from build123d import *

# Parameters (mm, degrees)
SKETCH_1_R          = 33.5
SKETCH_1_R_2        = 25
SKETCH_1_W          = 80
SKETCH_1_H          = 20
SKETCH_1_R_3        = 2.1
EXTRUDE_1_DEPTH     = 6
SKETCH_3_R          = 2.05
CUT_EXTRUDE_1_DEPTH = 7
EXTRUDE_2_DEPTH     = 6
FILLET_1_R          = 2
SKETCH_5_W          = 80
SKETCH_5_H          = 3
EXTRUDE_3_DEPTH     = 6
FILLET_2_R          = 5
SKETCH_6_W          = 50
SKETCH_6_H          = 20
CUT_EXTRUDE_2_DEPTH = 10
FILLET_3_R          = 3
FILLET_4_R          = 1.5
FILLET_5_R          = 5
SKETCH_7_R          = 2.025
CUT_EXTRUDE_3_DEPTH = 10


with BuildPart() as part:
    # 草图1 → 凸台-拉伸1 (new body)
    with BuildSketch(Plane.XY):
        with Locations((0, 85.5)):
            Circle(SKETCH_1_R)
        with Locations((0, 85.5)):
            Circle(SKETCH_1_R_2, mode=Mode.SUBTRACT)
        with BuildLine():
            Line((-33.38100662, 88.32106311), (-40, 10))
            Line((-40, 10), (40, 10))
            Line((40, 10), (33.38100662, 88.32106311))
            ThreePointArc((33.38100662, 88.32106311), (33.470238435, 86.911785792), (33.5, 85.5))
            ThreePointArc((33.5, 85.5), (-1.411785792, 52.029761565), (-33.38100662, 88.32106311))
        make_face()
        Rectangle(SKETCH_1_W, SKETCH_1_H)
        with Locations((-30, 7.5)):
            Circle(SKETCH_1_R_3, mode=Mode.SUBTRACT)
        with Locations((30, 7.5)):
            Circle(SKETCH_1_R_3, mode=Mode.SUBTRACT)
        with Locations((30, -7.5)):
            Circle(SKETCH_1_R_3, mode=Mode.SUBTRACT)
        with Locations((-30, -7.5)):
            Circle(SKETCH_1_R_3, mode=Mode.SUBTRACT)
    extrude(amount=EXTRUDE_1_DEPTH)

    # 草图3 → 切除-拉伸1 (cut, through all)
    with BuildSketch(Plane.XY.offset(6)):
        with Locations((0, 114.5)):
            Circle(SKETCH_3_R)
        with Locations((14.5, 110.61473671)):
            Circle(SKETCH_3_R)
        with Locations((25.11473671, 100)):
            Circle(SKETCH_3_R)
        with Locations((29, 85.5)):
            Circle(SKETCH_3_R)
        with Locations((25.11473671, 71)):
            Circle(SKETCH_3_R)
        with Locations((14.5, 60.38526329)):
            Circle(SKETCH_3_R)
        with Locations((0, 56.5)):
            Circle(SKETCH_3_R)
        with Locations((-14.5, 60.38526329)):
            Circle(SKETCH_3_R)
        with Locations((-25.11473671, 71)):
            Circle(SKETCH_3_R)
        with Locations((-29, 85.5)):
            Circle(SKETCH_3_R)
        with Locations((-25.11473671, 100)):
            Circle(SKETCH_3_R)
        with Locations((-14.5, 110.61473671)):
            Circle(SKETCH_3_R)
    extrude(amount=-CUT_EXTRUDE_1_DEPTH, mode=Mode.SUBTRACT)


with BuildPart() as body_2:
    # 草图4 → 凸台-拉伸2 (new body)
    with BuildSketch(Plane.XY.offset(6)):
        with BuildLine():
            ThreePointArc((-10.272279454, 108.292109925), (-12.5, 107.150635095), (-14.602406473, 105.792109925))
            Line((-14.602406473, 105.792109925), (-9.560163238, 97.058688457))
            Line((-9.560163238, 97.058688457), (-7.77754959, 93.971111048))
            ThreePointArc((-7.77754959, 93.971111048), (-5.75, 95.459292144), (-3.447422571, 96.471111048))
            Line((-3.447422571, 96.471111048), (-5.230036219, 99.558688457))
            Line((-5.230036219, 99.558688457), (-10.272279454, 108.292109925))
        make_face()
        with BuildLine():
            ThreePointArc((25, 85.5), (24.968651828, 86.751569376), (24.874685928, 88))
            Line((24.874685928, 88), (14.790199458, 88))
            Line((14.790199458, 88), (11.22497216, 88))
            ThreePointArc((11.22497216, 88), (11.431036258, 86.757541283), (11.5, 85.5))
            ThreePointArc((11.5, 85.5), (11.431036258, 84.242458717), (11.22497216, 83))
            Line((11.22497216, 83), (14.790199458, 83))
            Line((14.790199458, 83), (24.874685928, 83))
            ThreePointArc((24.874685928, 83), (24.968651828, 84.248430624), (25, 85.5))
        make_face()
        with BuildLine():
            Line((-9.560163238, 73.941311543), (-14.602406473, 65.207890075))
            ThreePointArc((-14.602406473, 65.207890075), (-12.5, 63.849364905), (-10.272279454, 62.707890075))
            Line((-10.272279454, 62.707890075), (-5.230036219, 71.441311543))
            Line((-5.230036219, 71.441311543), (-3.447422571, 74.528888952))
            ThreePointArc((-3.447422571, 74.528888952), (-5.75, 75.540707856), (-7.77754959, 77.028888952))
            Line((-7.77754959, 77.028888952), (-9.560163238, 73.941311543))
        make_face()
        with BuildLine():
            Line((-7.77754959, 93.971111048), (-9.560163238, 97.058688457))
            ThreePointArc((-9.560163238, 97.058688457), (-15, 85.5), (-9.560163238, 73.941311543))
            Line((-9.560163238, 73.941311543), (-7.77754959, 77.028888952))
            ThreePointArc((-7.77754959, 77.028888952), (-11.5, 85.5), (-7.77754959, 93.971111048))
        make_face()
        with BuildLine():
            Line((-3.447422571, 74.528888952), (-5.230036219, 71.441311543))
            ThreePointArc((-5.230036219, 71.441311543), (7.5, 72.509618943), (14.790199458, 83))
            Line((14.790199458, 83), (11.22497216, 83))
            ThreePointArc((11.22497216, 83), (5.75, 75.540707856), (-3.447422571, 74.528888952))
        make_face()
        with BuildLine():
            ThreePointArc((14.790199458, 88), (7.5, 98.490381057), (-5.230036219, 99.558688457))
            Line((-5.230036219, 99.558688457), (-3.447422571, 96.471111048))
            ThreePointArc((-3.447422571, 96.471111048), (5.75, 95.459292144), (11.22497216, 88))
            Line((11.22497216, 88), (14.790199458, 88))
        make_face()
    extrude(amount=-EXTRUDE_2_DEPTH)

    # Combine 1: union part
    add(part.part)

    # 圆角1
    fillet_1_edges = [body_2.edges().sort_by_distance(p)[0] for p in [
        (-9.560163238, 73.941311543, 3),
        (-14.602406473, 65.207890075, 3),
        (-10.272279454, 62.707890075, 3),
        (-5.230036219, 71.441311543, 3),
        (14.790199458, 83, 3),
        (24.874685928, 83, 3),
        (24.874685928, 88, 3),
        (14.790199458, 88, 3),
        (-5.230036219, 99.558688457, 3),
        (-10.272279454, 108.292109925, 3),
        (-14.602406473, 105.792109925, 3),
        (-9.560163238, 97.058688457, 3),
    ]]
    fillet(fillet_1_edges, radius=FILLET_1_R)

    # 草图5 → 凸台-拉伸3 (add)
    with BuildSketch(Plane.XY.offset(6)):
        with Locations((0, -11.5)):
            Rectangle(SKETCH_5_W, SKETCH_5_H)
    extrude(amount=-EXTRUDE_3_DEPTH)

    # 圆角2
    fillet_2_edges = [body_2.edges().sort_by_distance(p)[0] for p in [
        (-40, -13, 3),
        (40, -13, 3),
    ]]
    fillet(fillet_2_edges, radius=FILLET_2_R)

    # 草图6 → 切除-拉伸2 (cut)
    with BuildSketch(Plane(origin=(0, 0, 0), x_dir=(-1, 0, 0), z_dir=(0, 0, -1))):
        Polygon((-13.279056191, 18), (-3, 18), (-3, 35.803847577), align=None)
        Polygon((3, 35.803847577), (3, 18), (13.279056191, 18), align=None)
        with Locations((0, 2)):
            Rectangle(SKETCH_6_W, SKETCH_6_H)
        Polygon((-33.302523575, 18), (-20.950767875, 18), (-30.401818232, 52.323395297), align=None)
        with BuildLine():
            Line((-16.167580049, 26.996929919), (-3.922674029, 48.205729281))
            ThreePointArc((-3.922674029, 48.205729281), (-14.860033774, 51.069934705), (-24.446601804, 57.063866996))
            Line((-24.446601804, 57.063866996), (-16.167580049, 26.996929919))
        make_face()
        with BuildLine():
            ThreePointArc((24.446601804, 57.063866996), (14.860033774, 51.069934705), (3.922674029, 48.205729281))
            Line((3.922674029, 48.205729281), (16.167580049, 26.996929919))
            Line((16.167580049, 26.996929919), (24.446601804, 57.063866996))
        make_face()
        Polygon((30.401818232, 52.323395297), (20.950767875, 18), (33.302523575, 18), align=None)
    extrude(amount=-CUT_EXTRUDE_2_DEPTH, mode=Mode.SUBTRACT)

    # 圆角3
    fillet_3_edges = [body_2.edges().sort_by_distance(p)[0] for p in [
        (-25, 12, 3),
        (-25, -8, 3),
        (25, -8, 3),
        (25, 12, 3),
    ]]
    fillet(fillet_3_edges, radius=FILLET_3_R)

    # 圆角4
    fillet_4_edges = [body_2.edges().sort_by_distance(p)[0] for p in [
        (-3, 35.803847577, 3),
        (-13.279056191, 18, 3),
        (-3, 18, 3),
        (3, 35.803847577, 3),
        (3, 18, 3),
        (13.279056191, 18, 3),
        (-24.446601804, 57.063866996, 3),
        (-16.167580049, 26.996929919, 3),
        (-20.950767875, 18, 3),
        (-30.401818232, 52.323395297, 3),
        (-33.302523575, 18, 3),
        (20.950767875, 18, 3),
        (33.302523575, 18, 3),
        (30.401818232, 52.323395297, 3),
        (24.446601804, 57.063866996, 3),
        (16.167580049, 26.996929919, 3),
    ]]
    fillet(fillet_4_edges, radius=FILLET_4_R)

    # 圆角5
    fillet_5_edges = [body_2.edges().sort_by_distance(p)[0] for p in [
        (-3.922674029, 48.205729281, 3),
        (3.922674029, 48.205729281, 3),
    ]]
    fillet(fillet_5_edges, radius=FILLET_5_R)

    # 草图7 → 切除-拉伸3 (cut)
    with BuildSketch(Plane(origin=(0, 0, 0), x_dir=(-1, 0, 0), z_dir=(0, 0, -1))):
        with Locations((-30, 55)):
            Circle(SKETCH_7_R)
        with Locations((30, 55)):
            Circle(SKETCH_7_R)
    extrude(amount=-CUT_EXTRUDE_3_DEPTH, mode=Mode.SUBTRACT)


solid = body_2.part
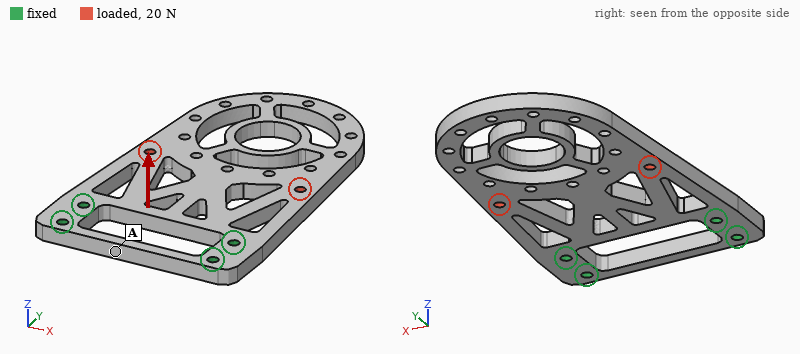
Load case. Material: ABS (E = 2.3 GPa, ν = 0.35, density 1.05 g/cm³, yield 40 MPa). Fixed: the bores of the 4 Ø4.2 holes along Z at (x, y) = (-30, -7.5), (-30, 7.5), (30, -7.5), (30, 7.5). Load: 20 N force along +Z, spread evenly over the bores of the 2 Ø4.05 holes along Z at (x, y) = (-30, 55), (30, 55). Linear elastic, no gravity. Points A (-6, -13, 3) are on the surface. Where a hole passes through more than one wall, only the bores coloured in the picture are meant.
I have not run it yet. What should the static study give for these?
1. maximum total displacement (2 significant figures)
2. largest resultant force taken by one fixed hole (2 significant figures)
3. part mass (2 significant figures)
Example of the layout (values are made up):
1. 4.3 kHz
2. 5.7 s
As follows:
1. 1.8 mm
2. 17 N
3. 34 g
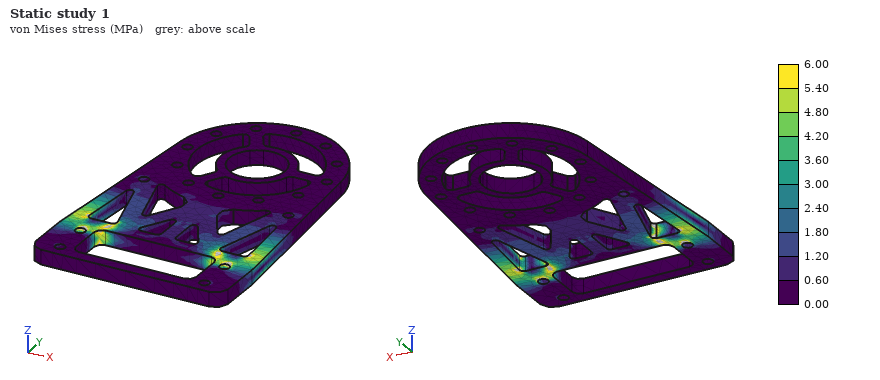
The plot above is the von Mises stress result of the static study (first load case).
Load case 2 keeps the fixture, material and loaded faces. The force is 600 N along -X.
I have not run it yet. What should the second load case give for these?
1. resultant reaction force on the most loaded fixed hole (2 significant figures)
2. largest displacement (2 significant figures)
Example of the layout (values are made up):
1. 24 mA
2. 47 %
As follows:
1. 490 N
2. 0.52 mm
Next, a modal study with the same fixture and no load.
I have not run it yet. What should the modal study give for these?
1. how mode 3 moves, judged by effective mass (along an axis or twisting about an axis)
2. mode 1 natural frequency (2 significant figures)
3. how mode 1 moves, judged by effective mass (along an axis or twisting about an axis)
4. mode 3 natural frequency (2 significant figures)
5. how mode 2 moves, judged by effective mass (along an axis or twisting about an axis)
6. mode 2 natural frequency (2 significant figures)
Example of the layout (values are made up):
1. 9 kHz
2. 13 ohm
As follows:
1. along Z
2. 110 Hz
3. along Z
4. 570 Hz
5. twisting about Y
6. 400 Hz
